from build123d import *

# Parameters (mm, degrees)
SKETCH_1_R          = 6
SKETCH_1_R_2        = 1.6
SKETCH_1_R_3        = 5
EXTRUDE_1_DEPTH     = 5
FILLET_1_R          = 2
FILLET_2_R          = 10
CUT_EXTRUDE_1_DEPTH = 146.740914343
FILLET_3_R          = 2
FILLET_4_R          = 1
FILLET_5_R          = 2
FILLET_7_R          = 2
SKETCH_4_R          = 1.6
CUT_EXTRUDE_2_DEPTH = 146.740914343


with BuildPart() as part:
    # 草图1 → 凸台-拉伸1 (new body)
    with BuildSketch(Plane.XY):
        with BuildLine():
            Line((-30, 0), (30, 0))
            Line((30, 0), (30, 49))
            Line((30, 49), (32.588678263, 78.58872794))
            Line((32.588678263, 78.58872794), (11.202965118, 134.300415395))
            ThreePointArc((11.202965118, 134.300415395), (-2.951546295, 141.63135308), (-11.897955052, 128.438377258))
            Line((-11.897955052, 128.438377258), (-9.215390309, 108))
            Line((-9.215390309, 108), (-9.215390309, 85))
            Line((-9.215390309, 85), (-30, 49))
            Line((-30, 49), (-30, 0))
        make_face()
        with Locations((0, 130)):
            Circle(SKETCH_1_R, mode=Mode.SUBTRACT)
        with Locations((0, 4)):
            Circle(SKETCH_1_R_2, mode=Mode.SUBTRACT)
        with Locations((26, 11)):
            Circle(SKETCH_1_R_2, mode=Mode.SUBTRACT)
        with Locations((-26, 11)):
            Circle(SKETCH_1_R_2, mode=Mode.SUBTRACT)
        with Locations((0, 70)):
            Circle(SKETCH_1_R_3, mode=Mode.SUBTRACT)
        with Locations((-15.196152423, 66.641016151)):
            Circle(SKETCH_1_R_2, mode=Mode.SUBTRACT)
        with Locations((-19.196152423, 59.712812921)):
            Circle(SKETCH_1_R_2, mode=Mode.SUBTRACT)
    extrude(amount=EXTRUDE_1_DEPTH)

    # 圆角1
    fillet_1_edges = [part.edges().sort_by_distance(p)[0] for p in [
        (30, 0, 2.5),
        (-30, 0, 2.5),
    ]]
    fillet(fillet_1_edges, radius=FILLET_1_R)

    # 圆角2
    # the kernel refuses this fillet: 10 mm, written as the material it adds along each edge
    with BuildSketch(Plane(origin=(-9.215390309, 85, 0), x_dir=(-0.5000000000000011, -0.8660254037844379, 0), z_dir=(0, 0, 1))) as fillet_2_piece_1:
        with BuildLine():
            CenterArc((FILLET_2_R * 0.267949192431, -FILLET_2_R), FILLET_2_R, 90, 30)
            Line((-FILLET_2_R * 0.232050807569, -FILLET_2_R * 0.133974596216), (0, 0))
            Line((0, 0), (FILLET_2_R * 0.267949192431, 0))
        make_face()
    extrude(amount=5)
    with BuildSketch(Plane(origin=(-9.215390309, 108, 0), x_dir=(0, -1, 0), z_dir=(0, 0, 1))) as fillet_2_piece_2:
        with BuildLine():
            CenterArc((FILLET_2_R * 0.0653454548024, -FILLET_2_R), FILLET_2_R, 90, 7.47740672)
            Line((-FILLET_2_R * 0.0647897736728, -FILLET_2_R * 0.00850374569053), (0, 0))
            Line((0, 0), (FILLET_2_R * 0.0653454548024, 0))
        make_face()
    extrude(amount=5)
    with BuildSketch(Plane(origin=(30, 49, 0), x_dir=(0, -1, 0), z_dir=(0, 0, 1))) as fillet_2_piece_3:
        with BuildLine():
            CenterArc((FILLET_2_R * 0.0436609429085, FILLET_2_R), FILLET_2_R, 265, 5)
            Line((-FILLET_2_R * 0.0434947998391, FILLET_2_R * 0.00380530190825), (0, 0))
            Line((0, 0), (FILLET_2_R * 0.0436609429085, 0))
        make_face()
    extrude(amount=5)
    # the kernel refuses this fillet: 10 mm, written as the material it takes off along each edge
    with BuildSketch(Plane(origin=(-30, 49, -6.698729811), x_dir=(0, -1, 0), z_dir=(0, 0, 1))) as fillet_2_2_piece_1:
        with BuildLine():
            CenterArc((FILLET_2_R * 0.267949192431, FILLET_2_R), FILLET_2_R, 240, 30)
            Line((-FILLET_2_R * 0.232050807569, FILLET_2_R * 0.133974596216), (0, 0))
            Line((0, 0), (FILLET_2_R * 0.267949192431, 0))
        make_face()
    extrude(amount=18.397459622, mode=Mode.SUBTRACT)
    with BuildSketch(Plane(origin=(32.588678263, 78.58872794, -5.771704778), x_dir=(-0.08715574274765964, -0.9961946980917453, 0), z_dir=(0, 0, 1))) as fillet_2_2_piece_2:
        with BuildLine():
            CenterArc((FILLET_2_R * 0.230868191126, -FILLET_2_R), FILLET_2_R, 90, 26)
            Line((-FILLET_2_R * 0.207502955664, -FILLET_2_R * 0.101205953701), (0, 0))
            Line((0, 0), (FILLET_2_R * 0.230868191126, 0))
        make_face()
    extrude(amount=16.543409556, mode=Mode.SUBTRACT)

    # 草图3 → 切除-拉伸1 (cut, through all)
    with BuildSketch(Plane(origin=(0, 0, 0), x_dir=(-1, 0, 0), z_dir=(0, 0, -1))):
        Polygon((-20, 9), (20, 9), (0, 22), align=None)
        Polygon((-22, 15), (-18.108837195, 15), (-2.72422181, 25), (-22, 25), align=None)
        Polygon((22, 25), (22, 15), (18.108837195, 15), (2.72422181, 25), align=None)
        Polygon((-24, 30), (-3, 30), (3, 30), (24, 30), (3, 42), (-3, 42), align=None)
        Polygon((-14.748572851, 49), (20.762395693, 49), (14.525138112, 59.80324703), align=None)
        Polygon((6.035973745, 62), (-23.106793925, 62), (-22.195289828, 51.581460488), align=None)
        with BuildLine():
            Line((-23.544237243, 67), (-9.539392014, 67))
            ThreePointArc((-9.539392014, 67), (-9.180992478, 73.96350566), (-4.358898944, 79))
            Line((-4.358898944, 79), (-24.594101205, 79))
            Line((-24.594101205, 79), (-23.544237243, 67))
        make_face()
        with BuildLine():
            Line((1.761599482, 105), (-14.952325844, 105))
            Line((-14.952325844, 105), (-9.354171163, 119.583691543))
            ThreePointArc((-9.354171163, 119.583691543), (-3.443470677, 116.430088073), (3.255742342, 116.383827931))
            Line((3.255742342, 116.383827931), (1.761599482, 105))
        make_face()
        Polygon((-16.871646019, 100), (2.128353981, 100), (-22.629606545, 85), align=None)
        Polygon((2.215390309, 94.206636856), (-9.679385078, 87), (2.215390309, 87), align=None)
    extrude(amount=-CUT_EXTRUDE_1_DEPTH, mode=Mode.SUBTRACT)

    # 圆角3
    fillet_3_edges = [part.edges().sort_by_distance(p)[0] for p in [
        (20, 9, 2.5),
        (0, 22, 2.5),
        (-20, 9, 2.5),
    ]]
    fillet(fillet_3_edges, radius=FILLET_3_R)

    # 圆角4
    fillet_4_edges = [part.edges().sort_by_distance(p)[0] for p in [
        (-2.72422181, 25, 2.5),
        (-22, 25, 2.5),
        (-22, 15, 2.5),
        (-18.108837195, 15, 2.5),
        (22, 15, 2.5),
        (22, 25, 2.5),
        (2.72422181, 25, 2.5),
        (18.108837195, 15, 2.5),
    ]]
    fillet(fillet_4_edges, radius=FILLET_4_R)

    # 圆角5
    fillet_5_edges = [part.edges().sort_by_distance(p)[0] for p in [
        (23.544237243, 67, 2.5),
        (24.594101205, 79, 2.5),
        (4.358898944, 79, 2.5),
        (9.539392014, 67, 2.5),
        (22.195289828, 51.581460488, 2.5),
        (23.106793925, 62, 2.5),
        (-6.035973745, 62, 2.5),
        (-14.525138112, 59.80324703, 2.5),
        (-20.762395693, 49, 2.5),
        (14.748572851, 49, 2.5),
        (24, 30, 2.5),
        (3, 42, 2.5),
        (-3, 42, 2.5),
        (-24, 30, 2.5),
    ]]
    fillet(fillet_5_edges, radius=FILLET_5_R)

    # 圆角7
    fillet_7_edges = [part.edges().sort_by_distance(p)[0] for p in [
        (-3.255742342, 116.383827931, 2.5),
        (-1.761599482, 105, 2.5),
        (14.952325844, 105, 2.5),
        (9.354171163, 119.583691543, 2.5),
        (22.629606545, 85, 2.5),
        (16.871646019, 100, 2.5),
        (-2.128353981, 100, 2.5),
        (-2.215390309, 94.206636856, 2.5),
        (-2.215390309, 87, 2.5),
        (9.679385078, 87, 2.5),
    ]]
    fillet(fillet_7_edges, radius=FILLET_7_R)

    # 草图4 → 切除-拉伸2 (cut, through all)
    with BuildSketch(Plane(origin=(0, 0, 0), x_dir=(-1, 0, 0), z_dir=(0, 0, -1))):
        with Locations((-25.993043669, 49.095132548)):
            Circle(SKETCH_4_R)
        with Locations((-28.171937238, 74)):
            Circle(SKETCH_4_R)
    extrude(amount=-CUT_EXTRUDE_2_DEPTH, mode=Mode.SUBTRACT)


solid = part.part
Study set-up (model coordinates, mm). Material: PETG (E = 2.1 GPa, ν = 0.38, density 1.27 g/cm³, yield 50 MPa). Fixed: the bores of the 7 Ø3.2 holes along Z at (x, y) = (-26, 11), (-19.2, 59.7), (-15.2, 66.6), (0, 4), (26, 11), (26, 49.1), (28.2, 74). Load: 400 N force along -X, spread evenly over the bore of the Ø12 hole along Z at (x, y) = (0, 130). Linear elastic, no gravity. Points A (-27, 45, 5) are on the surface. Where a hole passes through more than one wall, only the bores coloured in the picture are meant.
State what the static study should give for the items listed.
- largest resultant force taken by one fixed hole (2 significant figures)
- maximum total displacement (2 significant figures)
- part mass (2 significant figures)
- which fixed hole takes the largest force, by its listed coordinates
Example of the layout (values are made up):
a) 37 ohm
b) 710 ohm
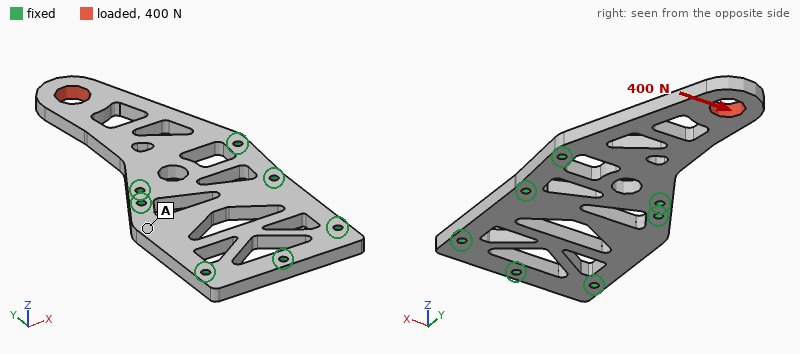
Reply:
a) 590 N
b) 1.6 mm
c) 29 g
d) (28.2, 74)
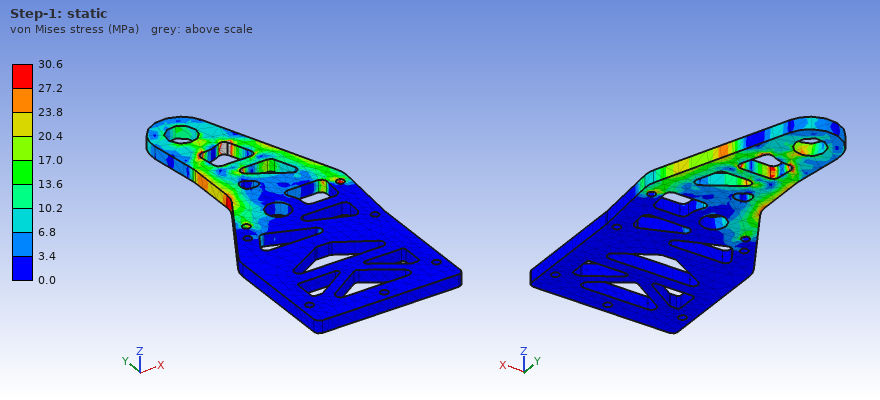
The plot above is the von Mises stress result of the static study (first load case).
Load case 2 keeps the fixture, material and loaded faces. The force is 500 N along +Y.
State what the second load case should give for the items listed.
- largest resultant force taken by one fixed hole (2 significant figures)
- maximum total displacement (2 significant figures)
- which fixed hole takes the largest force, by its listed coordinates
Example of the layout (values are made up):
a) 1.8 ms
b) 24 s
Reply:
a) 300 N
b) 0.50 mm
c) (-15.2, 66.6)
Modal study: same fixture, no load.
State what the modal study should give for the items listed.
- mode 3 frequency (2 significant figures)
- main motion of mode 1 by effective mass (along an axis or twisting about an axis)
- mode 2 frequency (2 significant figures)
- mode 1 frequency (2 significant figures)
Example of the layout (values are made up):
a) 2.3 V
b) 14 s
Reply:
a) 1100 Hz
b) along Z
c) 1000 Hz
d) 220 Hz
